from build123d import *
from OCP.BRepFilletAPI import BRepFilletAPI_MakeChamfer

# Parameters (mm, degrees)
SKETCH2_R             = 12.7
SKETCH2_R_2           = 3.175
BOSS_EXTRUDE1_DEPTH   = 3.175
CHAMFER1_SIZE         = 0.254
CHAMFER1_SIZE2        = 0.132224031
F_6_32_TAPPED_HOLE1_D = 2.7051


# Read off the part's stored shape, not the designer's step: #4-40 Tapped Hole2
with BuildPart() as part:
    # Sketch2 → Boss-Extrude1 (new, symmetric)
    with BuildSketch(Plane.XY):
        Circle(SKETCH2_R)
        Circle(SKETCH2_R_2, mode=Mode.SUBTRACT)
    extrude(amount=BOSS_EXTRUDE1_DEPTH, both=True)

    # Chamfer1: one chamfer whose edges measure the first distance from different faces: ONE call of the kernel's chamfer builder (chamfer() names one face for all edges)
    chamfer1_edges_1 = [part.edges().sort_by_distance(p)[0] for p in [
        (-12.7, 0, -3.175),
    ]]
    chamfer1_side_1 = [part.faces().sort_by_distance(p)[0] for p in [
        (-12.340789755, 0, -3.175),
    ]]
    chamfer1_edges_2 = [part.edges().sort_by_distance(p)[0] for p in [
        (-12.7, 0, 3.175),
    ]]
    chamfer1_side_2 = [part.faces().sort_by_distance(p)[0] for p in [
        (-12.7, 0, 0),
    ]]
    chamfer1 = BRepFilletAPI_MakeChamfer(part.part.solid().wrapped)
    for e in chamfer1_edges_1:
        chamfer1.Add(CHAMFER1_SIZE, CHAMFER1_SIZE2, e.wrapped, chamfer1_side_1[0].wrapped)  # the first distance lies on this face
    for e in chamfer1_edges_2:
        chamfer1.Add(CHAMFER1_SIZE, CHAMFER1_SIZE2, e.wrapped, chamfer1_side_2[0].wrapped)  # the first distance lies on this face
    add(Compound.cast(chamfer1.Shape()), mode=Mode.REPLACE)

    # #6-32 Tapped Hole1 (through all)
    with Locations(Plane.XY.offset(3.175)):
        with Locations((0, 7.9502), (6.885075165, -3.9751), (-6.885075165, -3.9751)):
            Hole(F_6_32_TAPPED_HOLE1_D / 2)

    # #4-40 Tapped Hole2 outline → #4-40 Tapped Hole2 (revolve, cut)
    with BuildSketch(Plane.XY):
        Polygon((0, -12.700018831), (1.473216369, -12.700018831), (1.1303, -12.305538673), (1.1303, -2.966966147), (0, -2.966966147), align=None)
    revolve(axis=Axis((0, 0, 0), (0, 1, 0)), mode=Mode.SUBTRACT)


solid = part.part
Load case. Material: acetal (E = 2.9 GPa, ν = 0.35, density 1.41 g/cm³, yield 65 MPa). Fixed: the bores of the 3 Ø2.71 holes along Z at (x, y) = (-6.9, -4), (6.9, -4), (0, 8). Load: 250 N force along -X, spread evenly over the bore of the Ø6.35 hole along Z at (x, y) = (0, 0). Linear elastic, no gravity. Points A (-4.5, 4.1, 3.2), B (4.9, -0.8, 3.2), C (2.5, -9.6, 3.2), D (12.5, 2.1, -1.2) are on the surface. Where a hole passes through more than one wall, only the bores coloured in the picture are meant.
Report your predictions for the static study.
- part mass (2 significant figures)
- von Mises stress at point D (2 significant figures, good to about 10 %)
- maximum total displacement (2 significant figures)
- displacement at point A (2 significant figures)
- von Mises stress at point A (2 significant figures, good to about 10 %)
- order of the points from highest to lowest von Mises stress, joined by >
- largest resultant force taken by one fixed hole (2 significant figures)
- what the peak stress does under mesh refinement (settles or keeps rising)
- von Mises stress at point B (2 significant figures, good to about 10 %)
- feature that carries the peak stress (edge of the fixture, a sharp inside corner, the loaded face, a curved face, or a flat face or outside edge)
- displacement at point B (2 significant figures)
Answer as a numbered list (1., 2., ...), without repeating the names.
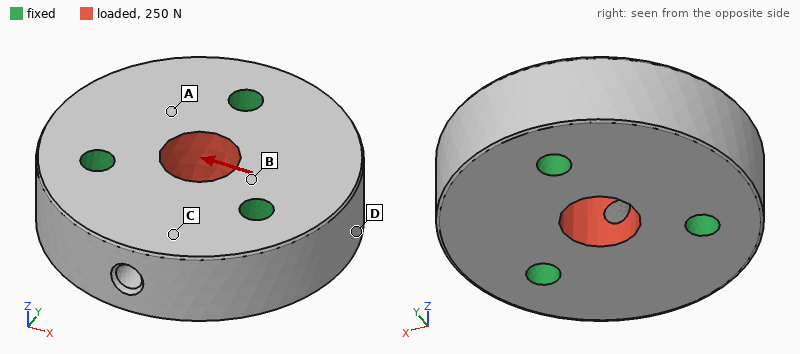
1. 4.0 g
2. 0.73 MPa
3. 6.3 µm
4. 4.2 µm
5. 1.4 MPa
6. B > A > D > C
7. 87 N
8. keeps rising
9. 2.1 MPa
10. edge of the fixture
11. 3.6 µm
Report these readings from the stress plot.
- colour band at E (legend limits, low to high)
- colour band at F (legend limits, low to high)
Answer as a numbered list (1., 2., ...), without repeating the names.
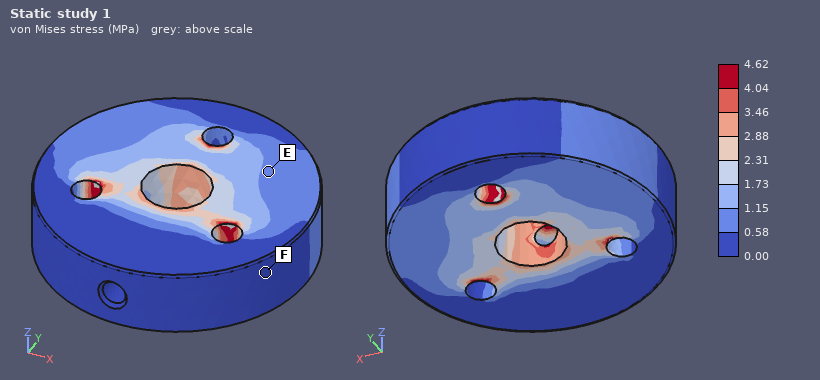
1. 0.58 to 1.15 MPa
2. 0.00 to 0.58 MPa
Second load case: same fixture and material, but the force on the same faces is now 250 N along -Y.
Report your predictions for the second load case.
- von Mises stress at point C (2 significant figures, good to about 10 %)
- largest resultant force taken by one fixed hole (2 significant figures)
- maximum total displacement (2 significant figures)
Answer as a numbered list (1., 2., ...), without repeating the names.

1. 0.97 MPa
2. 85 N
3. 6.8 µm
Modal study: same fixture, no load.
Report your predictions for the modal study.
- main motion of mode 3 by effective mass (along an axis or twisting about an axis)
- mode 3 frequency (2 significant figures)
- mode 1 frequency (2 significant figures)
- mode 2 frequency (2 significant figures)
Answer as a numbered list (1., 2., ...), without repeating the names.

1. along Z
2. 17 kHz
3. 15 kHz
4. 15 kHz
